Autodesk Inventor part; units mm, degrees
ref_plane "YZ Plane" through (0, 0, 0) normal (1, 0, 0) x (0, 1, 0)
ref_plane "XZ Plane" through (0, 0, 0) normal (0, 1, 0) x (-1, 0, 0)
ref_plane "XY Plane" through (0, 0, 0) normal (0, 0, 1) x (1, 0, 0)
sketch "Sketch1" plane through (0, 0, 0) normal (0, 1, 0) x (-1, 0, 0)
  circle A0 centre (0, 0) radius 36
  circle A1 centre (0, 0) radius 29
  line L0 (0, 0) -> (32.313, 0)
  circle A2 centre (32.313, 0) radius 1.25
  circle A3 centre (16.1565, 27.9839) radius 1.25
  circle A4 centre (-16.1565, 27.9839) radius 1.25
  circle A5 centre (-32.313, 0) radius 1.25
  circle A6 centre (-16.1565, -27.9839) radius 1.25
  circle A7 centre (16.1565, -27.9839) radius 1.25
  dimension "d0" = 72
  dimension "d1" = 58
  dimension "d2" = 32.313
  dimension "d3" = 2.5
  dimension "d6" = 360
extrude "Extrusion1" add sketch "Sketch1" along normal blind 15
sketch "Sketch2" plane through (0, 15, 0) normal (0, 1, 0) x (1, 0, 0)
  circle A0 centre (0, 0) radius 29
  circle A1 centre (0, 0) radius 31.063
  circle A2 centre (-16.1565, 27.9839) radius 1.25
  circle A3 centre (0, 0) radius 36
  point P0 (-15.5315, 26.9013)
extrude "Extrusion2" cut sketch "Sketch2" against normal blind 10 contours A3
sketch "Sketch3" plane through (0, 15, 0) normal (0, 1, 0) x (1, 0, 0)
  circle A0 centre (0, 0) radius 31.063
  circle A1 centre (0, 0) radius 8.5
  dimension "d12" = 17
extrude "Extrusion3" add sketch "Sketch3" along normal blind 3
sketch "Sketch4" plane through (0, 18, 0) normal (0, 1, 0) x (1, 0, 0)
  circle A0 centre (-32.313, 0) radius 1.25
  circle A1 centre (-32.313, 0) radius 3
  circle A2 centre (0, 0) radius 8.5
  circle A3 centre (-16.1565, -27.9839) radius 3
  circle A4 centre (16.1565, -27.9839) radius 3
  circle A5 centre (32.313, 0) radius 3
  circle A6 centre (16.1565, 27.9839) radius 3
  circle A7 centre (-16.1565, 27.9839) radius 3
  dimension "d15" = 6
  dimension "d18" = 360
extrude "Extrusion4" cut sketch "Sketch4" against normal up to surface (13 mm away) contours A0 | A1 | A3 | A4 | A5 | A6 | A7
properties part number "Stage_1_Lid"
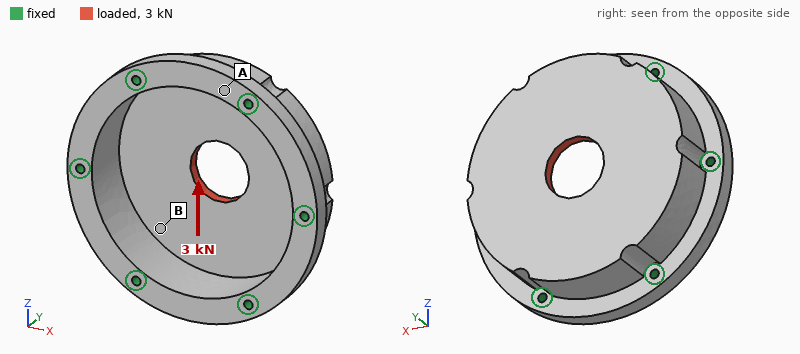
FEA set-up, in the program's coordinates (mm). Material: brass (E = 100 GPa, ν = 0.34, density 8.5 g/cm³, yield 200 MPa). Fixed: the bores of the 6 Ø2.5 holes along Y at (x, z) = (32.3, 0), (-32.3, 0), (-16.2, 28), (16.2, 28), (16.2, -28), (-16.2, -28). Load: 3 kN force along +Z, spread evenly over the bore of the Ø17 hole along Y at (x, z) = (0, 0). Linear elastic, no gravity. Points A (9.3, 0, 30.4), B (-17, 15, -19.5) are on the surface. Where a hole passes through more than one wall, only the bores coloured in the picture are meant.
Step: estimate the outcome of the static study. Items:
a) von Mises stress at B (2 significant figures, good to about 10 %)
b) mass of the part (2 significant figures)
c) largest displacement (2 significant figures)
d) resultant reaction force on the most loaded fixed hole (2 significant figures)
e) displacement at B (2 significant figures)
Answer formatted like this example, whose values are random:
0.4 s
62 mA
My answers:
24 MPa
160 g
17 µm
790 N
12 µm
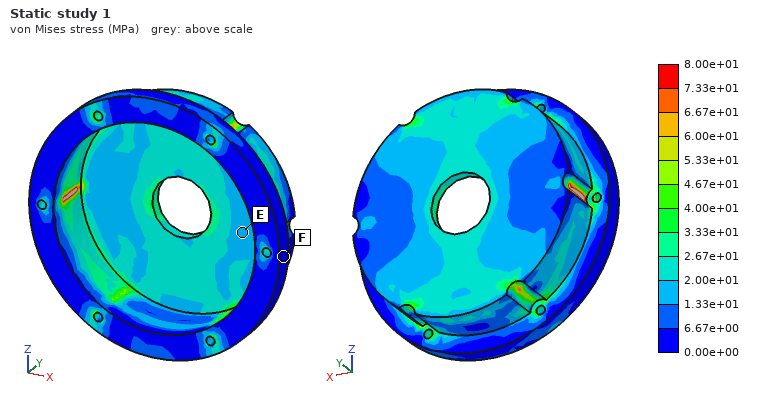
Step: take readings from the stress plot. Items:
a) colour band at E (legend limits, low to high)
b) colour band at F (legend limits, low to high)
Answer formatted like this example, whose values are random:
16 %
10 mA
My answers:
1.33e+01 to 2.00e+01 MPa
0.00e+00 to 6.67e+00 MPa
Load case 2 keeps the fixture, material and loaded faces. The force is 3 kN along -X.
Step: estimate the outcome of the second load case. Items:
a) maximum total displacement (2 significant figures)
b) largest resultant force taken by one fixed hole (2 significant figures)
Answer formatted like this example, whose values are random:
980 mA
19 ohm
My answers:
17 µm
720 N
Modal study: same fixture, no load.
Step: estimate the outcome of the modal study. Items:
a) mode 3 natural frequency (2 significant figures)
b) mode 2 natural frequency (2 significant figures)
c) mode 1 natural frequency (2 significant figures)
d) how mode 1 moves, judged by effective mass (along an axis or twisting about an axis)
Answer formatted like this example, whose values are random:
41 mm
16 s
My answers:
7900 Hz
7900 Hz
4200 Hz
along Y
